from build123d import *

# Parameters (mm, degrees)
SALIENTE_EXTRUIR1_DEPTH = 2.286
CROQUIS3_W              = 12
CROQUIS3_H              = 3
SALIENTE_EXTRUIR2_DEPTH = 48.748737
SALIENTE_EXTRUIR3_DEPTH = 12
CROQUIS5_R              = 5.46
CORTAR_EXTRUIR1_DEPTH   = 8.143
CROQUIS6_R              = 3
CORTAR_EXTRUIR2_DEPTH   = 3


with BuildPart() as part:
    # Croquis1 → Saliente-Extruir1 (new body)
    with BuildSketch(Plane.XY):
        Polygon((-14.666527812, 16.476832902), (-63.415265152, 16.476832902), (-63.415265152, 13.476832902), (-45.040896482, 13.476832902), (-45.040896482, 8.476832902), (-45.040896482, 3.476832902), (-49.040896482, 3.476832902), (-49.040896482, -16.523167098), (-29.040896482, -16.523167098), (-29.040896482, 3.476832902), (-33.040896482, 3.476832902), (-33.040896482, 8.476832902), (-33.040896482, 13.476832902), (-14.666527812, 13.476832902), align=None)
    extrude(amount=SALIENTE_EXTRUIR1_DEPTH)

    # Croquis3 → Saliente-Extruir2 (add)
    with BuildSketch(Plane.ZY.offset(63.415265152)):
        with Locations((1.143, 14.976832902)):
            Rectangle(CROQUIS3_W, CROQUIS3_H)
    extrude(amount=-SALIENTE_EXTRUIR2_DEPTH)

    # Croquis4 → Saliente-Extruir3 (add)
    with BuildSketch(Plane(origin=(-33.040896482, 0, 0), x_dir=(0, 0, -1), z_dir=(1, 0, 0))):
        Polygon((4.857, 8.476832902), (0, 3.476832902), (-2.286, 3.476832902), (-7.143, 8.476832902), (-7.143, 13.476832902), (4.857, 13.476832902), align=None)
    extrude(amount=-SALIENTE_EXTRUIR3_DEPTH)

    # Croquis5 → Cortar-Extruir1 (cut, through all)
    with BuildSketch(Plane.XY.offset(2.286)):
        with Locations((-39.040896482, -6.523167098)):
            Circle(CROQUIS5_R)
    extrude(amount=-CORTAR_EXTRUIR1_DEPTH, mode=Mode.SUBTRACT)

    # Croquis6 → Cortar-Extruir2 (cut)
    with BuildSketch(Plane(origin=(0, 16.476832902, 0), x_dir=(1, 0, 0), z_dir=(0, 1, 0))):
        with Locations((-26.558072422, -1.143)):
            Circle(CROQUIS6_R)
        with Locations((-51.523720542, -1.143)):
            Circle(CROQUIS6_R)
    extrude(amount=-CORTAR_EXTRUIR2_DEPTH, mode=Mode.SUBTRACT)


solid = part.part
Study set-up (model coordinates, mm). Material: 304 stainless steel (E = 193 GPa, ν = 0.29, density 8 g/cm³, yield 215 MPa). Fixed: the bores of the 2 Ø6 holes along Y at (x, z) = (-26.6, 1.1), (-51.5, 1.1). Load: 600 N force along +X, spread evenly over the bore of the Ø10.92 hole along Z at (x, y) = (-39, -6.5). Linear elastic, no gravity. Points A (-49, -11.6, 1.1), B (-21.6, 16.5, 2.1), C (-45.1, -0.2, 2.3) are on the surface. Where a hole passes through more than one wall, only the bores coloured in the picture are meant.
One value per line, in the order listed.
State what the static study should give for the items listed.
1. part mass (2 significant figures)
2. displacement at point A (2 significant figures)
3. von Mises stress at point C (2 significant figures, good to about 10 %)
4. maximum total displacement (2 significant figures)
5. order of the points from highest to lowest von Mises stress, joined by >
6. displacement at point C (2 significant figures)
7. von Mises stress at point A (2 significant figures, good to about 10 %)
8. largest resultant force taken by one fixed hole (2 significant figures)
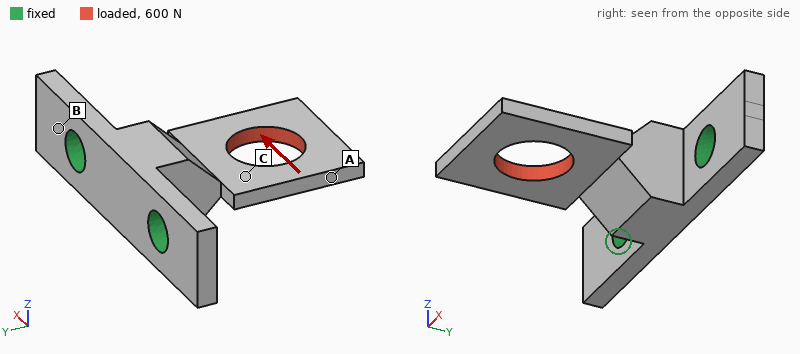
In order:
27 g
45 µm
42 MPa
53 µm
C > A > B
18 µm
32 MPa
840 N
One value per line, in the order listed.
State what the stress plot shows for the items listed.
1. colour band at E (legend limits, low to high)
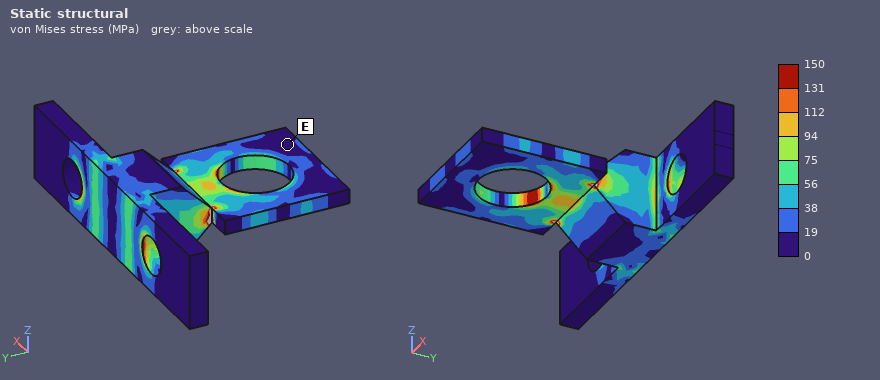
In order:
0 to 19 MPa
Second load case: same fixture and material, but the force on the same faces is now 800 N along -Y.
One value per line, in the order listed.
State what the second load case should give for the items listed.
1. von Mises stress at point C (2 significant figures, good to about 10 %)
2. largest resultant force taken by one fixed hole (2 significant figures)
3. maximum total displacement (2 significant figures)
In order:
38 MPa
430 N
8.0 µm
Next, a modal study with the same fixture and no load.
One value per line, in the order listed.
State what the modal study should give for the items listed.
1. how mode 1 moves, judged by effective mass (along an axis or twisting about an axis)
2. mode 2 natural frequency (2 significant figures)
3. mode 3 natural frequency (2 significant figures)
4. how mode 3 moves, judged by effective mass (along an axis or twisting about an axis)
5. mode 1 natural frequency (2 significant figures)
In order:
along Z
7300 Hz
8100 Hz
along X
3000 Hz
